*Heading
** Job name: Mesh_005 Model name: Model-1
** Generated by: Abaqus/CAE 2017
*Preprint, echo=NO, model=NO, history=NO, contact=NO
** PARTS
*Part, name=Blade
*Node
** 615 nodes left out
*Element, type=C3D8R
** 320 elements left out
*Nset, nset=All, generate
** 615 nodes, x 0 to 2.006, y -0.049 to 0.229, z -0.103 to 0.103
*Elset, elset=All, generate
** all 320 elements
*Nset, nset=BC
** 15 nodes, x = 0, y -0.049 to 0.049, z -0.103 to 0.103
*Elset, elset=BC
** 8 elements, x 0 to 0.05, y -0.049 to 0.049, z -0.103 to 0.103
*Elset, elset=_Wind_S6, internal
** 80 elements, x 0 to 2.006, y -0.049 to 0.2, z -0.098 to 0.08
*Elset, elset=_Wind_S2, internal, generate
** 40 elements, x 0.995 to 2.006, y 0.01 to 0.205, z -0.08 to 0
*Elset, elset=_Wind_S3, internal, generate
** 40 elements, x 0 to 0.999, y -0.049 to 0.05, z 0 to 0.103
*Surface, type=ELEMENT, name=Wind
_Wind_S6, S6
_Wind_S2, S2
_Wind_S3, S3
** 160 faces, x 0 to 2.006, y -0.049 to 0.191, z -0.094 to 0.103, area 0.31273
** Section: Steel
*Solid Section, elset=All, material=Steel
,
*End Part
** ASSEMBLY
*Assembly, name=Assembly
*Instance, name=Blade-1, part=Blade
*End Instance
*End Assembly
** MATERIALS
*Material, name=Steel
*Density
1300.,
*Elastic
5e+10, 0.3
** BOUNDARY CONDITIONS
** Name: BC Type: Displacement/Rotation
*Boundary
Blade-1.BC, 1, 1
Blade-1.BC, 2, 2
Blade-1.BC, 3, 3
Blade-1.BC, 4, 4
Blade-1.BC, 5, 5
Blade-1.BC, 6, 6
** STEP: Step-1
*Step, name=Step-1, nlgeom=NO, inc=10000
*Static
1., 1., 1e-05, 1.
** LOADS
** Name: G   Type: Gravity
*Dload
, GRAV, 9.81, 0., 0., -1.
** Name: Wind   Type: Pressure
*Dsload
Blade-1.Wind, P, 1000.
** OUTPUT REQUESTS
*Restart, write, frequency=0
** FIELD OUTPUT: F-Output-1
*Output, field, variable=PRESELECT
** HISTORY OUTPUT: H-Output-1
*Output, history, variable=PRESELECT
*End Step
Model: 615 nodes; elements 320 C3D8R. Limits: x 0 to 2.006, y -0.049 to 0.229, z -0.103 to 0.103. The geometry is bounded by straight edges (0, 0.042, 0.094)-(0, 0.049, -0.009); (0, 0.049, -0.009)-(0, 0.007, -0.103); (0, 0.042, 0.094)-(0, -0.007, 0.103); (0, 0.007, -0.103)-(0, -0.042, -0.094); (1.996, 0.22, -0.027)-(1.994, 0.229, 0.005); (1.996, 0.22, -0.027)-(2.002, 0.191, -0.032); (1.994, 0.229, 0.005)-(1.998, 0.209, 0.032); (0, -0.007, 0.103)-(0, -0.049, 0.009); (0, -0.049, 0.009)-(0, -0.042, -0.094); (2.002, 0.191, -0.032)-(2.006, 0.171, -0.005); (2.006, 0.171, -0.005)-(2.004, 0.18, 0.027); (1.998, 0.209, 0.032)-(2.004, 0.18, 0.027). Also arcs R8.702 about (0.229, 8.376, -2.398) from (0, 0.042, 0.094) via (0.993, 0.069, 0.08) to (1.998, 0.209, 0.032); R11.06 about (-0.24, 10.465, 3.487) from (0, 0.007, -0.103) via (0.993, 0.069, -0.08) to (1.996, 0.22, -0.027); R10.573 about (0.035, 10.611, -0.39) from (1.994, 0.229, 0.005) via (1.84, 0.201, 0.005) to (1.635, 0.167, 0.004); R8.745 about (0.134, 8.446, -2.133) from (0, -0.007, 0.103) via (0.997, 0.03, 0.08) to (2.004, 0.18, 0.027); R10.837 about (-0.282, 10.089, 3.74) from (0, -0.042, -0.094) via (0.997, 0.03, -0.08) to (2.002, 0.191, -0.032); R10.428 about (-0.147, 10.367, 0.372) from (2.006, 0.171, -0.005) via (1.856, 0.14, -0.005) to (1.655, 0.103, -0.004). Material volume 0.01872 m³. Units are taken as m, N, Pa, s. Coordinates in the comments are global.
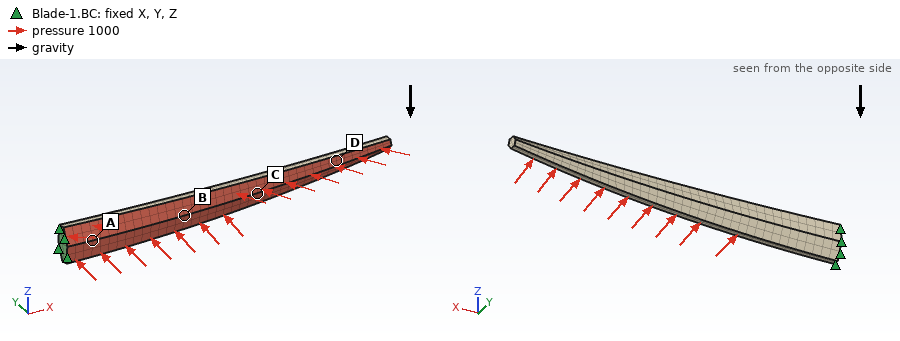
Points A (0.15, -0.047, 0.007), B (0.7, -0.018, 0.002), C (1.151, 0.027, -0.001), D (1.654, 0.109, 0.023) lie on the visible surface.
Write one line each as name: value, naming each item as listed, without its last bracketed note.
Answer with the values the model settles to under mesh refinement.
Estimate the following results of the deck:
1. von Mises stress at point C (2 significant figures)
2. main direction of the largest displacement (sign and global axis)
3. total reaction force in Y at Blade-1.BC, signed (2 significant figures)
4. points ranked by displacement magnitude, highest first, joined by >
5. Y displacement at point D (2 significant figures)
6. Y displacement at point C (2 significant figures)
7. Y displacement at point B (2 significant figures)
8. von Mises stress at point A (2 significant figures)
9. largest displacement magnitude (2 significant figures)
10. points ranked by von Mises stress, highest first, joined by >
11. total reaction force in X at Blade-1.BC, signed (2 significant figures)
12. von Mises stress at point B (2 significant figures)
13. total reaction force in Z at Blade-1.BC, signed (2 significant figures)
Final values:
von Mises stress at point C: 4.9e+05 Pa
main direction of the largest displacement: +Y
total reaction force in Y at Blade-1.BC, signed: -300 N
points ranked by displacement magnitude, highest first, joined by >: D > C > B > A
Y displacement at point D: 6.6e-04 m
Y displacement at point C: 3.6e-04 m
Y displacement at point B: 1.5e-04 m
von Mises stress at point A: 1.6e+06 Pa
largest displacement magnitude: 9.1e-04 m
points ranked by von Mises stress, highest first, joined by >: A > B > C > D
total reaction force in X at Blade-1.BC, signed: 29 N
von Mises stress at point B: 9.3e+05 Pa
total reaction force in Z at Blade-1.BC, signed: 250 N
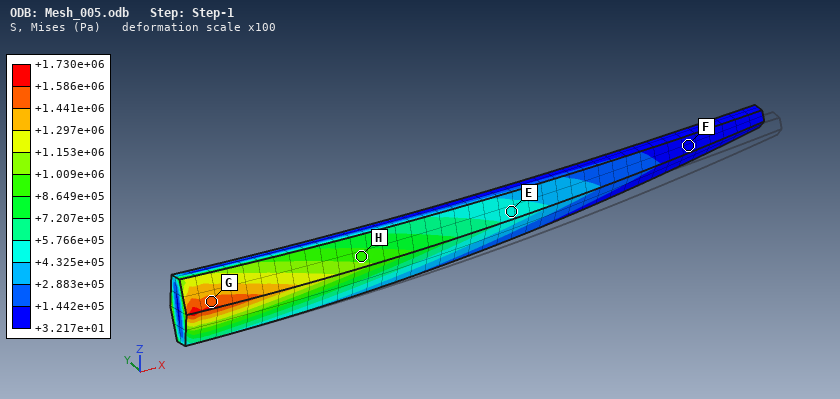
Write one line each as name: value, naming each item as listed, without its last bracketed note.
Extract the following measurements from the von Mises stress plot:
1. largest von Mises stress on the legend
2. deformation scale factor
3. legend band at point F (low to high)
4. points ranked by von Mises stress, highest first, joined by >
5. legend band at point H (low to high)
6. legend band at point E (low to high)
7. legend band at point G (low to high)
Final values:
largest von Mises stress on the legend: +1.730e+06 Pa
deformation scale factor: 100
legend band at point F: +3.217e+01 to +1.442e+05 Pa
points ranked by von Mises stress, highest first, joined by >: G > H > E > F
legend band at point H: +8.649e+05 to +1.009e+06 Pa
legend band at point E: +4.325e+05 to +5.766e+05 Pa
legend band at point G: +1.441e+06 to +1.586e+06 Pa
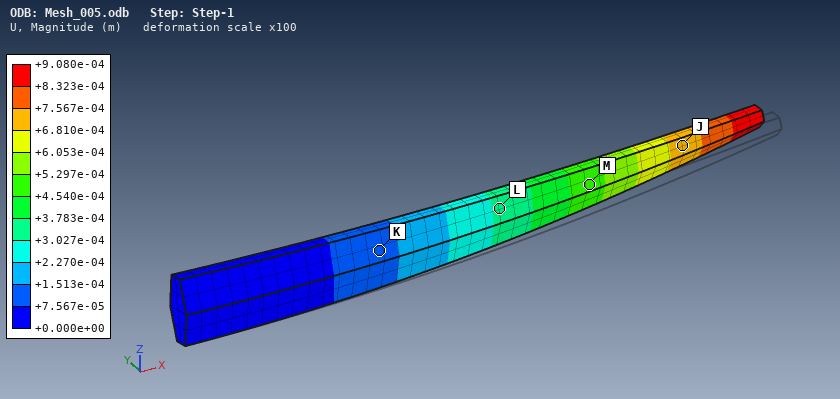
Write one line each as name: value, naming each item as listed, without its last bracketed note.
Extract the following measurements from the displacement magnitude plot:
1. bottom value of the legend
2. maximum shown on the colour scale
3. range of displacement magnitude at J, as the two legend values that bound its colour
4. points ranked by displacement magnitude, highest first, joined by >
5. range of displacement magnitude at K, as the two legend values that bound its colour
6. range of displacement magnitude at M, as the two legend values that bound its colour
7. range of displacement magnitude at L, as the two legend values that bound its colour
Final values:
bottom value of the legend: +0.000e+00 m
maximum shown on the colour scale: +9.080e-04 m
range of displacement magnitude at J, as the two legend values that bound its colour: +6.810e-04 to +7.567e-04 m
points ranked by displacement magnitude, highest first, joined by >: J > M > L > K
range of displacement magnitude at K, as the two legend values that bound its colour: +7.567e-05 to +1.513e-04 m
range of displacement magnitude at M, as the two legend values that bound its colour: +4.540e-04 to +5.297e-04 m
range of displacement magnitude at L, as the two legend values that bound its colour: +3.027e-04 to +3.783e-04 m
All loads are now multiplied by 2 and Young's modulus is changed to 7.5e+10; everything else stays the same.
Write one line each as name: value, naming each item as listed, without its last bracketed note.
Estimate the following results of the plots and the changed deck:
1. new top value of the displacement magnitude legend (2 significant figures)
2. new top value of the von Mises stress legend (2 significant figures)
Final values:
new top value of the displacement magnitude legend: 0.0012 m
new top value of the von Mises stress legend: 3.5e+06 Pa
